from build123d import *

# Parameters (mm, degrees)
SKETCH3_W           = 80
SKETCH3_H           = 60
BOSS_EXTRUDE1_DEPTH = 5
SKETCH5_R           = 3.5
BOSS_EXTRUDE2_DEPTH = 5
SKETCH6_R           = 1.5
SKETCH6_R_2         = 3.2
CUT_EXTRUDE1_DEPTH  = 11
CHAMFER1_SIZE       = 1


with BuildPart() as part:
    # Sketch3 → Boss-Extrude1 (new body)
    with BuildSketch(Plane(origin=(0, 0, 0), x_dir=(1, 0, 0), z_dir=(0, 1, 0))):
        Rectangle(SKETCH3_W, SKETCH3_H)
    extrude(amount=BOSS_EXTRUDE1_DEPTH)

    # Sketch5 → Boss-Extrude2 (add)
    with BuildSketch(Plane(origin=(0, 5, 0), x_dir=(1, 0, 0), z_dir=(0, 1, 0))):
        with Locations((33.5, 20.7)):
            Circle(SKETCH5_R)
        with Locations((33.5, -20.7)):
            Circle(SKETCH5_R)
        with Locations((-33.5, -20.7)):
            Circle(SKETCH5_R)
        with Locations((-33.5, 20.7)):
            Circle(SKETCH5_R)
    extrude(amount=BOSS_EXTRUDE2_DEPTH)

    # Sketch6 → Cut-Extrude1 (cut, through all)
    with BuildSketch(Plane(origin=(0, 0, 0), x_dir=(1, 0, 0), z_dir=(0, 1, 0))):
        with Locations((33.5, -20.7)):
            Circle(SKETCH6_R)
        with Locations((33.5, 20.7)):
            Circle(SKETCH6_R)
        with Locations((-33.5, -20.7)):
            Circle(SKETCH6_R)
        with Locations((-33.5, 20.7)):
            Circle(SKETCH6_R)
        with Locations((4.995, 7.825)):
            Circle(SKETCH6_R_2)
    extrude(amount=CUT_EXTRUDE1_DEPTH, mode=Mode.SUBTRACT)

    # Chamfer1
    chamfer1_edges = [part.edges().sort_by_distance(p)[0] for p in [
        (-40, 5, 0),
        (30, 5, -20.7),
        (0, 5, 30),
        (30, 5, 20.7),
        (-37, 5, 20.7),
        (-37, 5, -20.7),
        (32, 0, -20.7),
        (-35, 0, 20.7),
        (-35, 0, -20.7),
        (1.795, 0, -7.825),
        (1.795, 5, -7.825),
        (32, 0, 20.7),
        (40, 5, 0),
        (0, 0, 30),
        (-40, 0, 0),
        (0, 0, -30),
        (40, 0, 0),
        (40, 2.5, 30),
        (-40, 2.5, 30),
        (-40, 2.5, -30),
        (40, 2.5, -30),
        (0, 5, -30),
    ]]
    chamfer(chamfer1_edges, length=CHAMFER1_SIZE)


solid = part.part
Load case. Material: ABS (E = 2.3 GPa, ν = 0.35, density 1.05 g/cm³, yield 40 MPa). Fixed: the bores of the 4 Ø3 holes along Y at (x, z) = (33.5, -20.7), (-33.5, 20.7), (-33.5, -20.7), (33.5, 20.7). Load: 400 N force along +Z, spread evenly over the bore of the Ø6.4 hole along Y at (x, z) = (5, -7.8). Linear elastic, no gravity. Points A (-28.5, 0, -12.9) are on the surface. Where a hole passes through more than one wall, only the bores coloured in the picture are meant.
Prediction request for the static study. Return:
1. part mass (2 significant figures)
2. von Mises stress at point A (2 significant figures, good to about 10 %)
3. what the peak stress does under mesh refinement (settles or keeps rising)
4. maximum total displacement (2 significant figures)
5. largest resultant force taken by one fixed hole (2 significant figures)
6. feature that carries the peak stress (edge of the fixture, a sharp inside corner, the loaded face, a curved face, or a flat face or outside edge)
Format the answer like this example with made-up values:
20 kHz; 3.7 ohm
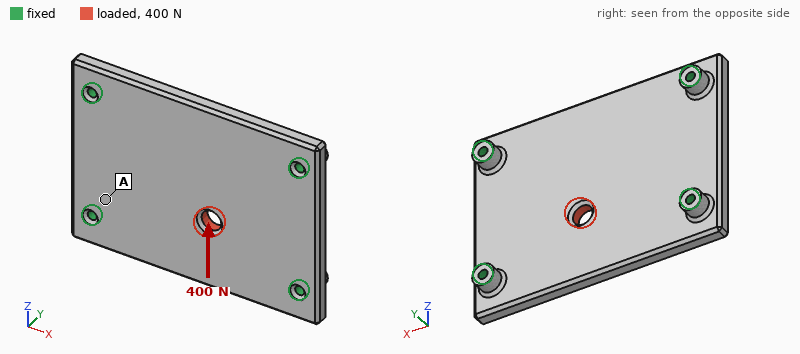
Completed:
25 g; 1.1 MPa; keeps rising; 51 µm; 130 N; edge of the fixture
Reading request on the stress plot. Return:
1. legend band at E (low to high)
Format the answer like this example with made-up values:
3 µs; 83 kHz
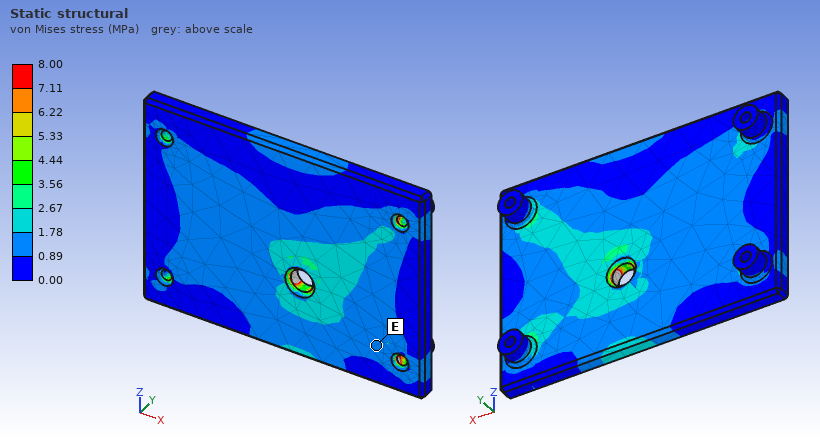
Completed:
0.89 to 1.78 MPa
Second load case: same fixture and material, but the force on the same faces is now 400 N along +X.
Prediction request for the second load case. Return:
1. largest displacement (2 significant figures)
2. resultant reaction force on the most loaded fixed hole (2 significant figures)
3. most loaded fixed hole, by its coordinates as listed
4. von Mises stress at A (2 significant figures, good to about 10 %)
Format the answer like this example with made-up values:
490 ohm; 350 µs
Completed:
33 µm; 140 N; (33.5, -20.7); 0.86 MPa
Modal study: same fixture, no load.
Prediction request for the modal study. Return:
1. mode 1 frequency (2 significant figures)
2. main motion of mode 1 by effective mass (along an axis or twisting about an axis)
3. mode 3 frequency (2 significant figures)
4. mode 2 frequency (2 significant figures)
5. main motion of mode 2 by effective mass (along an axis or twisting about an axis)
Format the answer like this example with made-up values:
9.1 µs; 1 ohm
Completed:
1500 Hz; along Y; 3100 Hz; 2000 Hz; twisting about X
